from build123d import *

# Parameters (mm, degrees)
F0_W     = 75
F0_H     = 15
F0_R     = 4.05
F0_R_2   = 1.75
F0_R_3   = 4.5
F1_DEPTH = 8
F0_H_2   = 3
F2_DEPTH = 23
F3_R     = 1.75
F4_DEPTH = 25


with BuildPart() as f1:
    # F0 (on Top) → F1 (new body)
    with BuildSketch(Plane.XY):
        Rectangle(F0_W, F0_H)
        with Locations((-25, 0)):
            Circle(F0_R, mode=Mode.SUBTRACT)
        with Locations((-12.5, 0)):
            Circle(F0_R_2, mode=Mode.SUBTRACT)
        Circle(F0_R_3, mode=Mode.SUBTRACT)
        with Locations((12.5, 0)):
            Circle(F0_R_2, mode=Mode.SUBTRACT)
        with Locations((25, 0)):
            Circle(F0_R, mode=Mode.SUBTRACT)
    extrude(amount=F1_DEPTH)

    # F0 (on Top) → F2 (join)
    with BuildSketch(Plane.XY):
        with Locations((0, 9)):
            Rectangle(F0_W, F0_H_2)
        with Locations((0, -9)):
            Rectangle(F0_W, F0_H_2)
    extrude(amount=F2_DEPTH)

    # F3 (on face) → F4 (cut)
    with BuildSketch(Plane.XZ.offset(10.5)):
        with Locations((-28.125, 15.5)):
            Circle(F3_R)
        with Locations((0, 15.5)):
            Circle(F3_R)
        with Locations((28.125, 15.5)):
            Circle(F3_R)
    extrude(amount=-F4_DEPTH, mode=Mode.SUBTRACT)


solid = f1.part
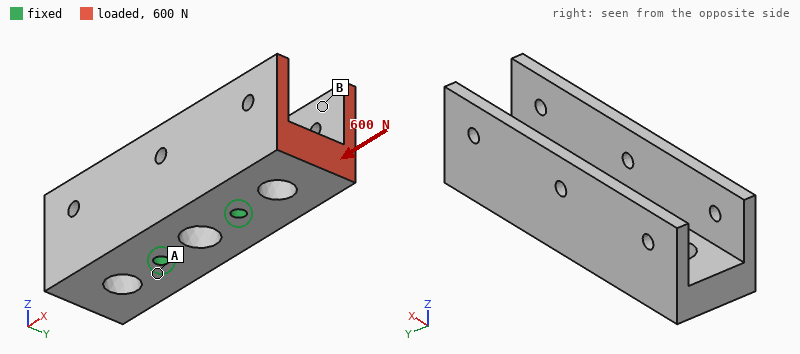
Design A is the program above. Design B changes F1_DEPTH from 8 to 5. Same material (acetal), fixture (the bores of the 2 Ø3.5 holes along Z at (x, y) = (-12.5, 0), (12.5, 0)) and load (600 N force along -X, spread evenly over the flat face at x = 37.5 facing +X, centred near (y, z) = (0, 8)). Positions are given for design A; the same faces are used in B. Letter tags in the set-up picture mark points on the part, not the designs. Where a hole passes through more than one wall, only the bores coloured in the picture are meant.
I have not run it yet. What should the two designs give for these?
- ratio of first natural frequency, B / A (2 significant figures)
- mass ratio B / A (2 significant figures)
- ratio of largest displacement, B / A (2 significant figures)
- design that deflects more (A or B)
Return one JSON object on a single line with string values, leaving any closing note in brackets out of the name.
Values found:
{"ratio of first natural frequency, B / A": "0.64", "mass ratio B / A": "0.84", "ratio of largest displacement, B / A": "2.1", "design that deflects more": "B"}
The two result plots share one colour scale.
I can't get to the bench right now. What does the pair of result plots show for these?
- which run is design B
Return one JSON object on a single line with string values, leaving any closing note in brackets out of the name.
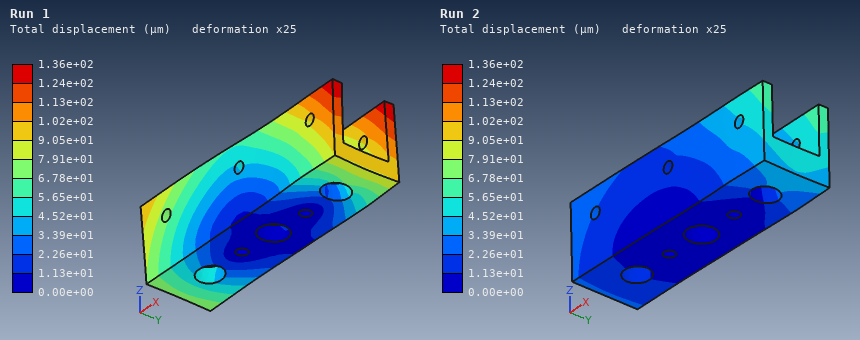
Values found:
{"which run is design B": "Run 1"}
